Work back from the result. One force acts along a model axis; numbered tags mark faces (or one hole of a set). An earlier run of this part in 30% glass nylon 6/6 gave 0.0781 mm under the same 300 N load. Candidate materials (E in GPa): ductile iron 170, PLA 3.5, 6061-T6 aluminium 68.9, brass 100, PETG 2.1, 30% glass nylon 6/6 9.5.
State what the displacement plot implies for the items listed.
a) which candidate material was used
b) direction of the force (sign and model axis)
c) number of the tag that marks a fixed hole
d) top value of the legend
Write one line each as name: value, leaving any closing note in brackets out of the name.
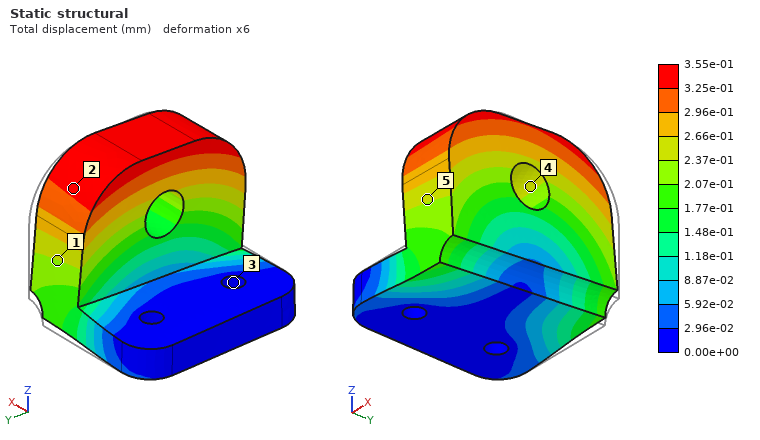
which candidate material was used: PETG
direction of the force: -Y
number of the tag that marks a fixed hole: 3
top value of the legend: 3.55e-01 mm
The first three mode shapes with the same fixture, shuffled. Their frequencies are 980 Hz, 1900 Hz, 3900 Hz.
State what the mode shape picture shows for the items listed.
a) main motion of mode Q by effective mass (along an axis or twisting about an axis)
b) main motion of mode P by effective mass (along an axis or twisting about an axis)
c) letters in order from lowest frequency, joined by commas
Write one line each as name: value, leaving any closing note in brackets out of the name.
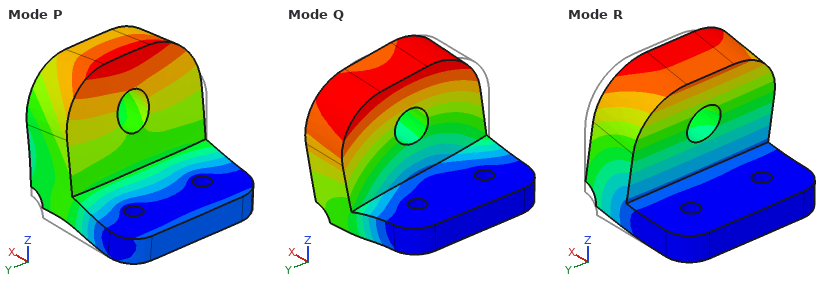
main motion of mode Q by effective mass: along Y
main motion of mode P by effective mass: along Z
letters in order from lowest frequency, joined by commas: R, Q, P
